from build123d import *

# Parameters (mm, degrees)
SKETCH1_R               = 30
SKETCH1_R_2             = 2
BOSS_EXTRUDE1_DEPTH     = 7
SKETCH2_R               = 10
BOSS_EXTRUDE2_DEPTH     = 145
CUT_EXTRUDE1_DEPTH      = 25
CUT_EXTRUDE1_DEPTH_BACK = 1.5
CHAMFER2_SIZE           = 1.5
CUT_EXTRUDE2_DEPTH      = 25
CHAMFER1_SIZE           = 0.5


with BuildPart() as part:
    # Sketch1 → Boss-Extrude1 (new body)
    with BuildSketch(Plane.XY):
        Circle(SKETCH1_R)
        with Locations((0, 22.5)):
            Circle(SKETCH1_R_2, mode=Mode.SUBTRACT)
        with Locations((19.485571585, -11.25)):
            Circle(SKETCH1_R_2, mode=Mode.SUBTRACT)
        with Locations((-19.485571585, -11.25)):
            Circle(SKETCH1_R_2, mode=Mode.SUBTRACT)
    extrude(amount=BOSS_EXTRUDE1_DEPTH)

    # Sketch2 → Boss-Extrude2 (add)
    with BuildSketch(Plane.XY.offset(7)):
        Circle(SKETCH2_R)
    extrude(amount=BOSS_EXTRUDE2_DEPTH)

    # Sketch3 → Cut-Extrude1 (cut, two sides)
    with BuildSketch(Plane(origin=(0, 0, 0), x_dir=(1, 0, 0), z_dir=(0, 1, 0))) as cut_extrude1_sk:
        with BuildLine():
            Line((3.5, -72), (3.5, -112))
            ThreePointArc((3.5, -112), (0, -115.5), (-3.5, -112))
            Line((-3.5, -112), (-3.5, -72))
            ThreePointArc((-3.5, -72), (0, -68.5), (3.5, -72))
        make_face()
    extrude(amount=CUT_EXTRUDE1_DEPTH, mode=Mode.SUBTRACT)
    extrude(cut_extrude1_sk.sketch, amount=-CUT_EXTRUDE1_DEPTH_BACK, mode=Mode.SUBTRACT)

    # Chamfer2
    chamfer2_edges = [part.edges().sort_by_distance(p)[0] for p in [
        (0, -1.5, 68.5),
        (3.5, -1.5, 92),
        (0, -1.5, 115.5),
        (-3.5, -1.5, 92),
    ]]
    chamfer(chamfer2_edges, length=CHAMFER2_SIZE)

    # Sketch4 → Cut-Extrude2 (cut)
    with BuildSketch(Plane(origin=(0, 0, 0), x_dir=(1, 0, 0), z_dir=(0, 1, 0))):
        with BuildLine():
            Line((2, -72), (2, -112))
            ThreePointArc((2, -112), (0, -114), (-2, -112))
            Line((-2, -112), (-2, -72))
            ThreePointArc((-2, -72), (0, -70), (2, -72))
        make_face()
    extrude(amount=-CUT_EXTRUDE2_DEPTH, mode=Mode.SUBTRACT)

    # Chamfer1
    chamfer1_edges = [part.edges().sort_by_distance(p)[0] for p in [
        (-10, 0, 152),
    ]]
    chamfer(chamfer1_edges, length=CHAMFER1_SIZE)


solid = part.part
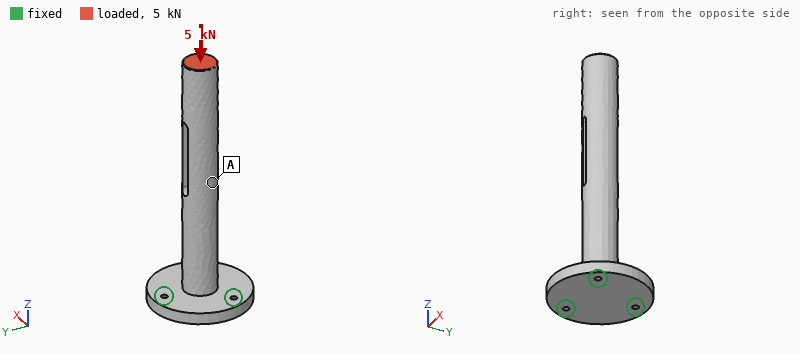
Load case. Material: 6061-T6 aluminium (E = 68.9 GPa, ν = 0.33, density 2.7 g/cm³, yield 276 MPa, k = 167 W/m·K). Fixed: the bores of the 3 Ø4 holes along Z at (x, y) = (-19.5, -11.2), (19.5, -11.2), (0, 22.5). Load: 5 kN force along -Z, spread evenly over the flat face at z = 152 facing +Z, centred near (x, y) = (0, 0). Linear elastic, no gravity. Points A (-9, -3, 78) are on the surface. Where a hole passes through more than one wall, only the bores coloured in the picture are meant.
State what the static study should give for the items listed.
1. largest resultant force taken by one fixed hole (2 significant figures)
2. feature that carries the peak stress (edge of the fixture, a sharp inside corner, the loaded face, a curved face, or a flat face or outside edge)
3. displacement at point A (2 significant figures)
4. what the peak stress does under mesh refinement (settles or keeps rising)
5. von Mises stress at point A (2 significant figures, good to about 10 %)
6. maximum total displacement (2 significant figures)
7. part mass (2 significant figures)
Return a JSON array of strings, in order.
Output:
["1.7 kN", "edge of the fixture", "39 µm", "keeps rising", "19 MPa", "76 µm", "160 g"]
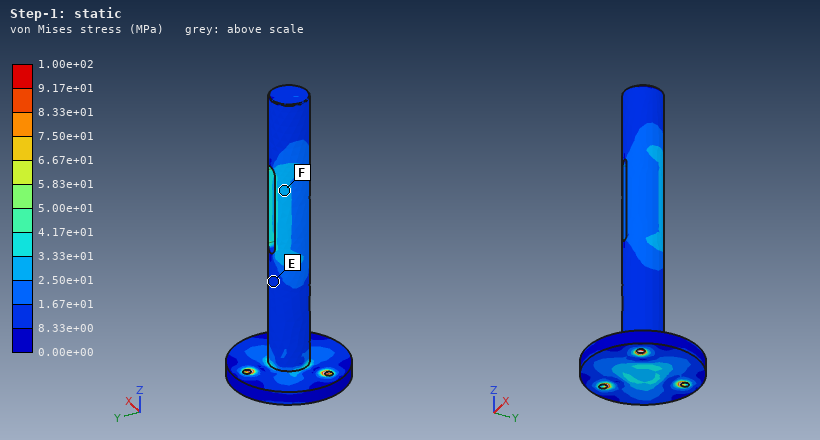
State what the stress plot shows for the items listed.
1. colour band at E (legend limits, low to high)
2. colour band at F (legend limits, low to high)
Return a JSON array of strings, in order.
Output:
["8.33e+00 to 1.67e+01 MPa", "2.50e+01 to 3.33e+01 MPa"]
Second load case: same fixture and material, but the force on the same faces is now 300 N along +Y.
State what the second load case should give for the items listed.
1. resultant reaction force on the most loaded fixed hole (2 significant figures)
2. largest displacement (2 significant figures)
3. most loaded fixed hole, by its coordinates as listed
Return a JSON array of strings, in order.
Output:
["1.3 kN", "0.84 mm", "(0, 22.5)"]
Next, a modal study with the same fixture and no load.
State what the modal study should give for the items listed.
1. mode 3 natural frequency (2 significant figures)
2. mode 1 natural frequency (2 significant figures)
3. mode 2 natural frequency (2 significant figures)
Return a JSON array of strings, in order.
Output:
["3100 Hz", "560 Hz", "570 Hz"]
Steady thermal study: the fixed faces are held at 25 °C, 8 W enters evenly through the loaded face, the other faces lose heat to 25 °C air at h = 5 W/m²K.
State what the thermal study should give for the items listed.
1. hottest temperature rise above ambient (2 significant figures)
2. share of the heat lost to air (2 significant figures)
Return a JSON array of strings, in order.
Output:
["26 K", "9.3 %"]
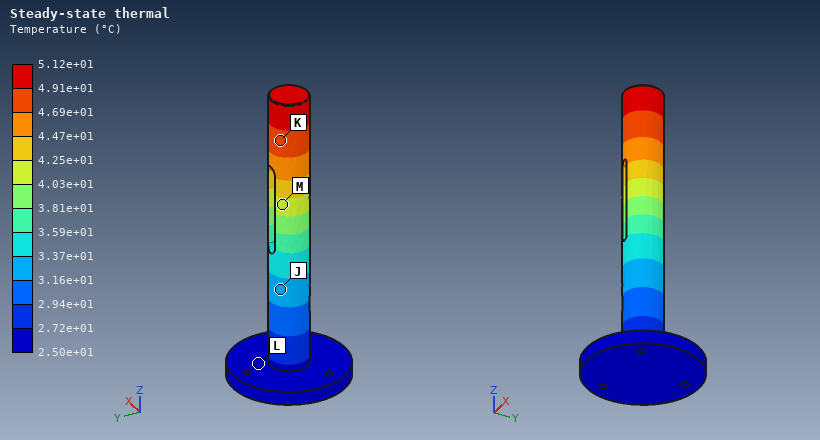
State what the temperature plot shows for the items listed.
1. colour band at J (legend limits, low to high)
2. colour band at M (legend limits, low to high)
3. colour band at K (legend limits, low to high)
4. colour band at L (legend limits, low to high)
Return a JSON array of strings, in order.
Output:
["3.16e+01 to 3.37e+01 °C", "4.03e+01 to 4.25e+01 °C", "4.69e+01 to 4.91e+01 °C", "2.50e+01 to 2.72e+01 °C"]
